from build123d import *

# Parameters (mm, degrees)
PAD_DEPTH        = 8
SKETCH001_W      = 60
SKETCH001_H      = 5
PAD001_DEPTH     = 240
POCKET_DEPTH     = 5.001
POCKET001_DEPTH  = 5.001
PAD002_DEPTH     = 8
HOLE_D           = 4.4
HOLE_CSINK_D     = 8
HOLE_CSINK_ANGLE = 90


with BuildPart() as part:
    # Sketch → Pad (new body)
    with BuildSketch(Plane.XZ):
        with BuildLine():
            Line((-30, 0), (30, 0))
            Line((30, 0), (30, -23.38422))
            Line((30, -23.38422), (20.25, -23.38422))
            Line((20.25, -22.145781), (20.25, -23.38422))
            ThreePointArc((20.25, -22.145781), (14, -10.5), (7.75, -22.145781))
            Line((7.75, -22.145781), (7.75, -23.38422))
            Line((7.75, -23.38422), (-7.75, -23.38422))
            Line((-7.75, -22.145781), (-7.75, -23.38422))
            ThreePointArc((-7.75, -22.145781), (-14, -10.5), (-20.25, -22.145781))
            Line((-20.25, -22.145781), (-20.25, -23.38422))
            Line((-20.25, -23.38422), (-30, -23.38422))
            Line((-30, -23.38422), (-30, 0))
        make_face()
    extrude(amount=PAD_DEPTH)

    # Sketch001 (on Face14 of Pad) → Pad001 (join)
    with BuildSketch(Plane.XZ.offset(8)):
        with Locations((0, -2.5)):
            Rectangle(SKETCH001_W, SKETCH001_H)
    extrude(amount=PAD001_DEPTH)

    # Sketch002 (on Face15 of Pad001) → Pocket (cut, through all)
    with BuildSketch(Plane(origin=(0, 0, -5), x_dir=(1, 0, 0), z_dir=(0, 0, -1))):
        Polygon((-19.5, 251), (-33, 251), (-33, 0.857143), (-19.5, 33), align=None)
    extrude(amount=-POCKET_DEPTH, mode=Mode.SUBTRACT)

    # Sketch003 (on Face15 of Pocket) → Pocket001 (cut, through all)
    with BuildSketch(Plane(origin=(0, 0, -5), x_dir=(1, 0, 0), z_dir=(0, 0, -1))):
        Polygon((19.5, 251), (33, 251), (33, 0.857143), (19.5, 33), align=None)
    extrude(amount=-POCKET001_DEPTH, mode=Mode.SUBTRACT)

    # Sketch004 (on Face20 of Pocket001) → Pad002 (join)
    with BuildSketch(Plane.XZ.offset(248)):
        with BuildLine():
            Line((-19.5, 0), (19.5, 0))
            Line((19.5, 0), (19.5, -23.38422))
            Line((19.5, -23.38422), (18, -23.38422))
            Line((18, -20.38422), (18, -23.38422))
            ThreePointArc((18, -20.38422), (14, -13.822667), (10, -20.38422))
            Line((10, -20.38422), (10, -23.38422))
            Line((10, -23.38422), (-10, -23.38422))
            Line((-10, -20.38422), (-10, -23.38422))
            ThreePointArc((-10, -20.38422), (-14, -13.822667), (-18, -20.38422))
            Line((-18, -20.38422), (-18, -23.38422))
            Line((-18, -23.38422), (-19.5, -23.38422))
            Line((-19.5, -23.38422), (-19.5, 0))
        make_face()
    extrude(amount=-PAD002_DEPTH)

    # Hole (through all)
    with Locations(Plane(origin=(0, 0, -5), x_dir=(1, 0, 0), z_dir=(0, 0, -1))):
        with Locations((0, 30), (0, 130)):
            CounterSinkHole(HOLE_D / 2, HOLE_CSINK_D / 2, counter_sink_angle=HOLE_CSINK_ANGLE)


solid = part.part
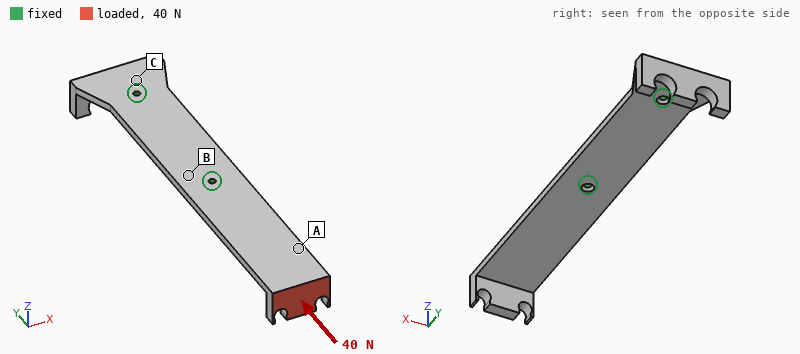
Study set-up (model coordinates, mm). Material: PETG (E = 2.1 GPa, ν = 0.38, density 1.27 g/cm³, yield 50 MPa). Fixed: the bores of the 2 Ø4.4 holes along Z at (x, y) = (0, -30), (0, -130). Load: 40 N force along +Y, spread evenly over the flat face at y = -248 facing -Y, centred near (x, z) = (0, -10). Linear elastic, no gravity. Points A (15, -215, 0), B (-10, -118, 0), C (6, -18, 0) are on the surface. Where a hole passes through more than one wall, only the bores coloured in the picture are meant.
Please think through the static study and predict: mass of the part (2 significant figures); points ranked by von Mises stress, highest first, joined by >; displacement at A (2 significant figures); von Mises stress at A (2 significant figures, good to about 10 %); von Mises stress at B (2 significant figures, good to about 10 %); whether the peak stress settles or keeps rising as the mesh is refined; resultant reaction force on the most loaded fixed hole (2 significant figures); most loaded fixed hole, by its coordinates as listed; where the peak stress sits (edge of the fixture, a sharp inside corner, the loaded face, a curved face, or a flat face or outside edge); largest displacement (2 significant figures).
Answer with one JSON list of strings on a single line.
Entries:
["78 g", "A > B > C", "1.5 mm", "1.7 MPa", "0.43 MPa", "keeps rising", "28 N", "(0, -130)", "edge of the fixture", "2.9 mm"]
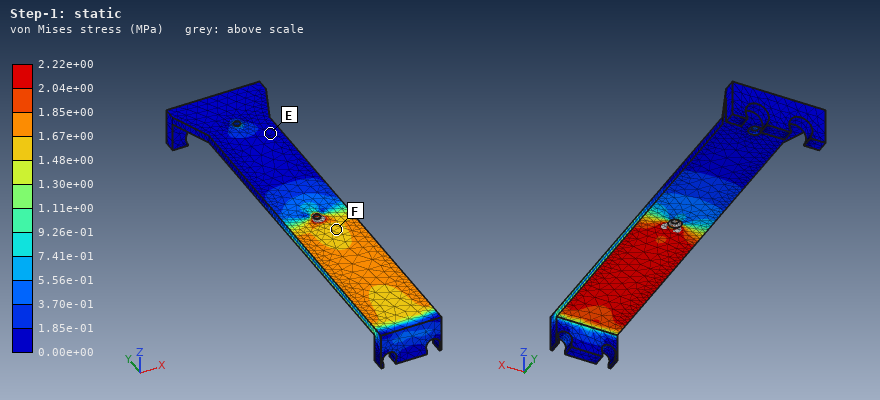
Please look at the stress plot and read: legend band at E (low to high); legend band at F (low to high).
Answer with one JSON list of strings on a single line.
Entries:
["0.00e+00 to 1.85e-01 MPa", "1.48e+00 to 1.67e+00 MPa"]
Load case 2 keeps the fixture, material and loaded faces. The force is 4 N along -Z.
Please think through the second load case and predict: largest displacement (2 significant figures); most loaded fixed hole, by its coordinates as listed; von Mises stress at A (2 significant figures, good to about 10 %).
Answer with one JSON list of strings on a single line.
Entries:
["3.0 mm", "(0, -130)", "0.84 MPa"]
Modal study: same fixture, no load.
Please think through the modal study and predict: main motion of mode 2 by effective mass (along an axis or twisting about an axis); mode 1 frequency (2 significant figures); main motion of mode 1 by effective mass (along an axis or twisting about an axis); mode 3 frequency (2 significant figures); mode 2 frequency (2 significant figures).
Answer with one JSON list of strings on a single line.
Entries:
["along X", "53 Hz", "along Z", "340 Hz", "260 Hz"]
